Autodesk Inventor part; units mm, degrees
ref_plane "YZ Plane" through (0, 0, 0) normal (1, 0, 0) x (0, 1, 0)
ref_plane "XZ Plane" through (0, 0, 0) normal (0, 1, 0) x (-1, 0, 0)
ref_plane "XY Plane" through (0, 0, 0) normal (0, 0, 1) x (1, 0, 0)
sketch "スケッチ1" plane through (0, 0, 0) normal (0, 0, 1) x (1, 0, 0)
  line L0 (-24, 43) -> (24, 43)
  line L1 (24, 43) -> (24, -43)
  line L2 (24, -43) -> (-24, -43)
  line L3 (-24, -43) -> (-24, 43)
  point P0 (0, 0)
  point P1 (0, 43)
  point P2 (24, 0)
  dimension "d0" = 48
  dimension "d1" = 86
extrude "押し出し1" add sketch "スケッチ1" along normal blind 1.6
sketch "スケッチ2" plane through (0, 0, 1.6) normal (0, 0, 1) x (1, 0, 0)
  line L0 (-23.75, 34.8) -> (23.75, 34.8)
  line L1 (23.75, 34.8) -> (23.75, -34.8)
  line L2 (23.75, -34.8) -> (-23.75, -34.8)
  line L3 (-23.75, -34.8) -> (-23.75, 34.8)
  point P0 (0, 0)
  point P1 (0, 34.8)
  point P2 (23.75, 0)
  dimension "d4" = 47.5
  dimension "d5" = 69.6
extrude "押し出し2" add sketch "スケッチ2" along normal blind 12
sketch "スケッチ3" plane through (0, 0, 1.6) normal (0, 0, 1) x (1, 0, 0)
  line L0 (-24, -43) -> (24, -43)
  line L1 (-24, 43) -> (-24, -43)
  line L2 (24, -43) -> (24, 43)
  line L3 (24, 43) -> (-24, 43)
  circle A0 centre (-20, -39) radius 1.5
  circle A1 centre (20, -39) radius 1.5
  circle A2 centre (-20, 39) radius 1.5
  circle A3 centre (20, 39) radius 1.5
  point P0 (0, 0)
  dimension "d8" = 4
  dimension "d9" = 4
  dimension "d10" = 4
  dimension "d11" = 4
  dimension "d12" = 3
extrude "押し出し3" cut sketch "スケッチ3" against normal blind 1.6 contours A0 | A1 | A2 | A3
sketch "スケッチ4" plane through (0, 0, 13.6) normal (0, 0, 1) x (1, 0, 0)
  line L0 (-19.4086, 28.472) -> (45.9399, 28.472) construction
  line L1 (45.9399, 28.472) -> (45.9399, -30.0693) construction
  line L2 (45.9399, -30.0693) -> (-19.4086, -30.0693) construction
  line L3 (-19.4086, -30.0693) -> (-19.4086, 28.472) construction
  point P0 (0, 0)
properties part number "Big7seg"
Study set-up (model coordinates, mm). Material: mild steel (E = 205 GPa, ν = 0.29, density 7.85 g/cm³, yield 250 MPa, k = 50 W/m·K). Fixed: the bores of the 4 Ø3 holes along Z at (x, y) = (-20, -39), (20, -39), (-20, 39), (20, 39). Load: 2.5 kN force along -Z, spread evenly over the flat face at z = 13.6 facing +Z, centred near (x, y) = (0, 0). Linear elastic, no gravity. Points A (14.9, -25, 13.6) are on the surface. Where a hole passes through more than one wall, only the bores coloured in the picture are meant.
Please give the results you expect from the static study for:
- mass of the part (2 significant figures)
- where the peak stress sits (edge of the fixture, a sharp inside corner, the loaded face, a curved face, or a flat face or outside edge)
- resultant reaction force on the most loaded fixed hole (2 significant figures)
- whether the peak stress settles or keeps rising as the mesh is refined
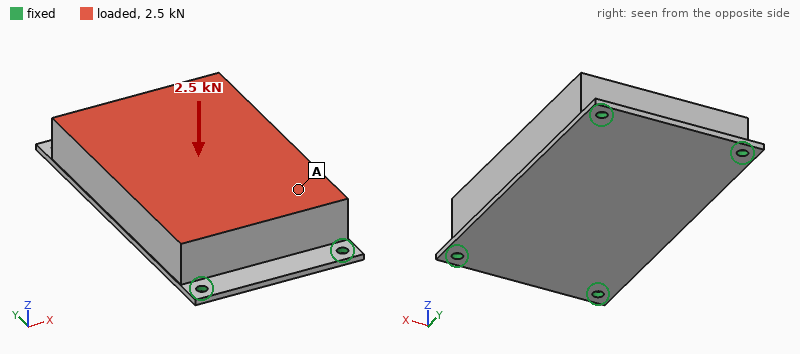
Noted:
360 g
edge of the fixture
850 N
keeps rising
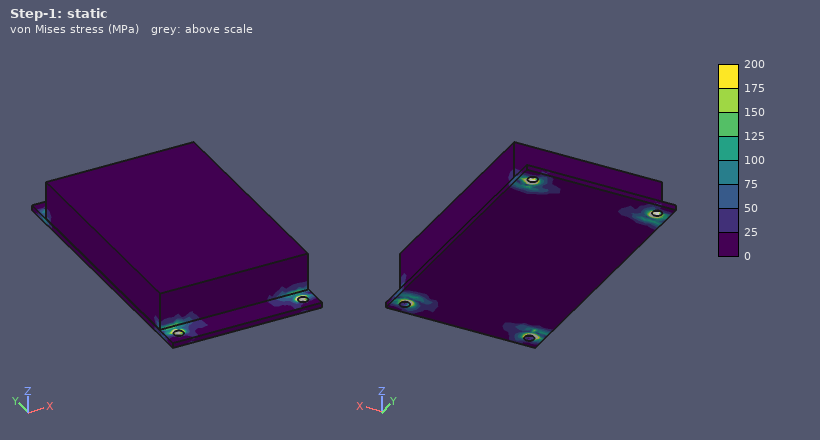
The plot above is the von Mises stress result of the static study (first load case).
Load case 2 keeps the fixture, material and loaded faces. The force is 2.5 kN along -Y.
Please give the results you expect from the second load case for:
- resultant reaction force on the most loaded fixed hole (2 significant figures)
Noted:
680 N
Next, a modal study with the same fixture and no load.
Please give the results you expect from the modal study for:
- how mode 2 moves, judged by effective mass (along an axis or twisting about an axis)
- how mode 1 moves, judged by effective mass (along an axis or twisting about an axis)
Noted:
along X
along Z
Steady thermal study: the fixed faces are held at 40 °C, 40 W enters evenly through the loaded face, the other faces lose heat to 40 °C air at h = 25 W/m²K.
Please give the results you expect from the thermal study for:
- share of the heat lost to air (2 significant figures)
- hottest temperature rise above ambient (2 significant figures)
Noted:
24 %
59 K
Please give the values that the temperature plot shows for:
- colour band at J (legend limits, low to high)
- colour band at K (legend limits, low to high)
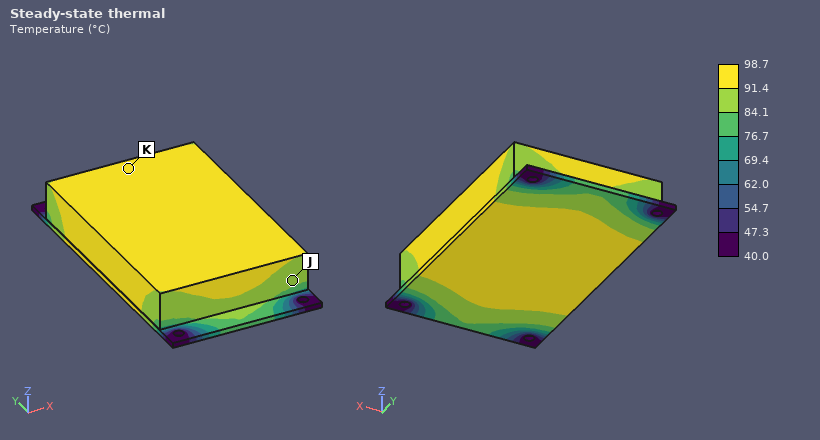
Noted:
84.1 to 91.4 °C
91.4 to 98.7 °C
